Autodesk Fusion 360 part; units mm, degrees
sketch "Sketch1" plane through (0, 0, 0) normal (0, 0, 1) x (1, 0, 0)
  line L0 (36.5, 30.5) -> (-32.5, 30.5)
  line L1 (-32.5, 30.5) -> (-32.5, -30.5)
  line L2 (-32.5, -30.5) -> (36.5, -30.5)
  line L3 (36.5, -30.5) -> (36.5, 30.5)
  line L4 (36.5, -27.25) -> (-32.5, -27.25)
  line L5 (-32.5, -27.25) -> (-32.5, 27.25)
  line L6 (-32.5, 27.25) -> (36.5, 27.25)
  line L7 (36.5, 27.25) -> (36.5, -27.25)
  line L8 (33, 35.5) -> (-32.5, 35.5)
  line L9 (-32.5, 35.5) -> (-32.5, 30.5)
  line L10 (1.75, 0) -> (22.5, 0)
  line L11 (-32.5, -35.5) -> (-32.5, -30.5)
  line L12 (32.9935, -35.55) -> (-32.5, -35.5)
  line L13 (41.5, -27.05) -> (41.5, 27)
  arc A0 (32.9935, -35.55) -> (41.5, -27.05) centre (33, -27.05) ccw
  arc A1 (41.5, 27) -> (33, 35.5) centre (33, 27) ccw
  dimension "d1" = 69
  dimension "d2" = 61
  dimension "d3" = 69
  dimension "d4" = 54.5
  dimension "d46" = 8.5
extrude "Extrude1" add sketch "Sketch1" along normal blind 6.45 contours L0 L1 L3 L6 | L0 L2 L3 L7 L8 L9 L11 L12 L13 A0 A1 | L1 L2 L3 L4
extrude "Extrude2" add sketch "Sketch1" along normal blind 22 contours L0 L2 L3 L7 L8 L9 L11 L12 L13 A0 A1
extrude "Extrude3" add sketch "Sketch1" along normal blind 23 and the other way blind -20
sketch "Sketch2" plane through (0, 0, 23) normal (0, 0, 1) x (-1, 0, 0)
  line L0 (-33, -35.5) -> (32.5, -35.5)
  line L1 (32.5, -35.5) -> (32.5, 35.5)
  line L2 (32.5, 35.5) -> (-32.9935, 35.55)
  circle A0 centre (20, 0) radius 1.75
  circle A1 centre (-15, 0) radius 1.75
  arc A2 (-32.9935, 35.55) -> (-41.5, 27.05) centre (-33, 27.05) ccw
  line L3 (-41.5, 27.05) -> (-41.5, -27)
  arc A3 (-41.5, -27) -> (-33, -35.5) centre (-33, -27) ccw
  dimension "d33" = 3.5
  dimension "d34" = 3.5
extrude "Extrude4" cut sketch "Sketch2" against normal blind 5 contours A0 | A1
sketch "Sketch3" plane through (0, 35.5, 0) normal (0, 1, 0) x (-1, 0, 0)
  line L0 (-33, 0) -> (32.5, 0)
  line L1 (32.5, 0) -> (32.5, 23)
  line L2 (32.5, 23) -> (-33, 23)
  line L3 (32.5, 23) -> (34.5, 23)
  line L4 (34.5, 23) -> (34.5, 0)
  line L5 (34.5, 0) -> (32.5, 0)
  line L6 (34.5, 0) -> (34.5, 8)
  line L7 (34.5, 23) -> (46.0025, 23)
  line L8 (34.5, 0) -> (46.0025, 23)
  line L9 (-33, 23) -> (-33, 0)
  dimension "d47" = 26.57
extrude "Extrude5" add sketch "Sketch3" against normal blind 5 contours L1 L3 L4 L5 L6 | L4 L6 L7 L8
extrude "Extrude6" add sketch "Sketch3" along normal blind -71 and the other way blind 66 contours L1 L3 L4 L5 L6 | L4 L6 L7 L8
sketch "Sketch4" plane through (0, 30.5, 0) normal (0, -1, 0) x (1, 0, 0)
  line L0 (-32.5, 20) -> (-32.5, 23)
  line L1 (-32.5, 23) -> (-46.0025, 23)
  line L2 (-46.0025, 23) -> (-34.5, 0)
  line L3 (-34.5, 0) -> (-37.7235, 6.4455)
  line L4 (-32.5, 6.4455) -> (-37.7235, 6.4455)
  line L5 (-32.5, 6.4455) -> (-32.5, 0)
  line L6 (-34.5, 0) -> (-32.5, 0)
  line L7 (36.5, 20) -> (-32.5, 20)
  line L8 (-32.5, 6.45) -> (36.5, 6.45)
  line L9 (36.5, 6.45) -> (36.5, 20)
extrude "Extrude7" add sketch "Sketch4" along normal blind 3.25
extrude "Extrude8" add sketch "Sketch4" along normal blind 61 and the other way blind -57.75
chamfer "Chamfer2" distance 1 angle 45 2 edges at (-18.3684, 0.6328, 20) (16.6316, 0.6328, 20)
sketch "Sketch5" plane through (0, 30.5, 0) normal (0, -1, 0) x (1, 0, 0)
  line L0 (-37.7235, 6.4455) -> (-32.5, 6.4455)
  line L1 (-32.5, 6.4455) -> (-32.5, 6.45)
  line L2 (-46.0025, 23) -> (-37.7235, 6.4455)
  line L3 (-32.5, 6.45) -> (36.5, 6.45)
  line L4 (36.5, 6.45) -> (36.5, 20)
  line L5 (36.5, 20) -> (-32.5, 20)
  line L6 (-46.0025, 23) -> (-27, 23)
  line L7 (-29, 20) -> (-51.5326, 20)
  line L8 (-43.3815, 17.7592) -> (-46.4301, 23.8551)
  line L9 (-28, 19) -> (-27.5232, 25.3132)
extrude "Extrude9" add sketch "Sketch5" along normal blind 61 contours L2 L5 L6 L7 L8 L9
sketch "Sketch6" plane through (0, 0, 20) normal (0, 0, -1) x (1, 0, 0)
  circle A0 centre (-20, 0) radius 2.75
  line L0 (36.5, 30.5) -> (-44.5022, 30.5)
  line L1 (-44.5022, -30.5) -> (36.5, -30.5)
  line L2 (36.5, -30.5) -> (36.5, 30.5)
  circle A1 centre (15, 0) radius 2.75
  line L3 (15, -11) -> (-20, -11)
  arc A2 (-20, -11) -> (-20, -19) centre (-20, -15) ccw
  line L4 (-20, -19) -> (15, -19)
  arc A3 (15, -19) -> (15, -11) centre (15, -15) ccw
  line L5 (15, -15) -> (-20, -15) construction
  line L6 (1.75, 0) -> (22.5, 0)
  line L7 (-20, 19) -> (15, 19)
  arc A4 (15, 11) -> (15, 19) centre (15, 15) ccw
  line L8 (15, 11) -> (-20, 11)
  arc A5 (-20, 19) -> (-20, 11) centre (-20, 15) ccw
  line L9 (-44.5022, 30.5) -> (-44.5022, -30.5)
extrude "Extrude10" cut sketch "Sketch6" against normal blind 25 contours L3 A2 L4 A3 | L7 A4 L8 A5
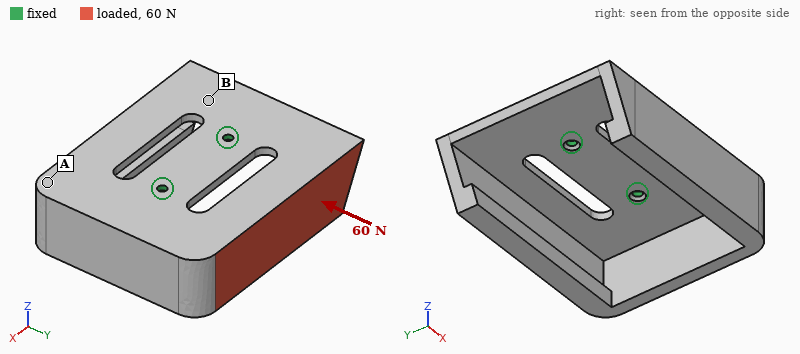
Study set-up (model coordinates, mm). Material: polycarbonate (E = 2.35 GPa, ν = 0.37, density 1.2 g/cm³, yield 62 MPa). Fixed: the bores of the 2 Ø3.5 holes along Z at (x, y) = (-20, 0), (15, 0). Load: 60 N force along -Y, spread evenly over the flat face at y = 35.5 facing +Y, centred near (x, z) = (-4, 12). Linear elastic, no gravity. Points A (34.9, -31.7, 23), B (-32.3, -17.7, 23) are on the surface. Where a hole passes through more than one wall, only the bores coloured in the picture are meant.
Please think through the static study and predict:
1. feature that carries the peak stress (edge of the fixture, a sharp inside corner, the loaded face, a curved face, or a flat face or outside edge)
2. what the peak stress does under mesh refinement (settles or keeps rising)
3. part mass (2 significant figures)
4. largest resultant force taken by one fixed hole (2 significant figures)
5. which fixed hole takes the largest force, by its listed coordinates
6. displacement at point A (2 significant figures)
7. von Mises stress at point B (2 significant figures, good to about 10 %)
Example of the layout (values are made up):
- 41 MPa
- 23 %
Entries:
- edge of the fixture
- keeps rising
- 49 g
- 33 N
- (-20, 0)
- 0.90 mm
- 2.7 MPa
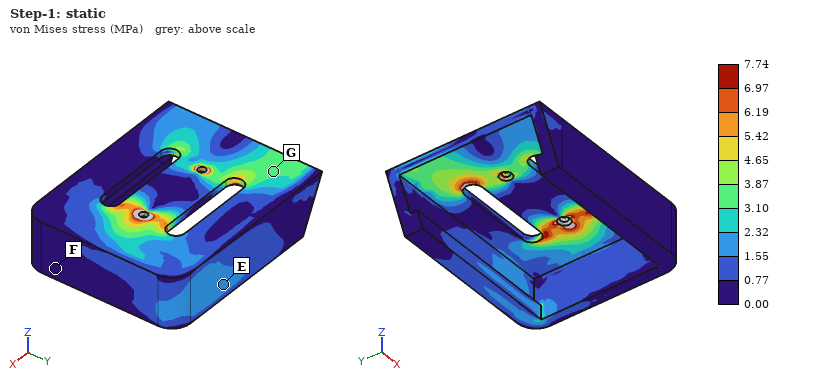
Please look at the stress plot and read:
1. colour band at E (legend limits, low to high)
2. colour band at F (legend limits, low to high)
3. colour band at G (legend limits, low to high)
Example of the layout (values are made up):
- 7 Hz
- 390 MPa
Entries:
- 1.55 to 2.32 MPa
- 0.00 to 0.77 MPa
- 3.10 to 3.87 MPa
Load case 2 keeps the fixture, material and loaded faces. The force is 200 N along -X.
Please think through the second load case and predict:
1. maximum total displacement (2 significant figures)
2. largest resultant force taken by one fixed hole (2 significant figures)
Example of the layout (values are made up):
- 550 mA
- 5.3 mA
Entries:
- 1.2 mm
- 220 N
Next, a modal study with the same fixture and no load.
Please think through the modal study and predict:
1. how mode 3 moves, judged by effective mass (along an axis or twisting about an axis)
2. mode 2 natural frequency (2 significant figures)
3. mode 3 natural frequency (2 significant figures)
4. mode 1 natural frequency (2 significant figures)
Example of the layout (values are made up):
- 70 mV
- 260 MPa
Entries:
- along Z
- 300 Hz
- 360 Hz
- 130 Hz
